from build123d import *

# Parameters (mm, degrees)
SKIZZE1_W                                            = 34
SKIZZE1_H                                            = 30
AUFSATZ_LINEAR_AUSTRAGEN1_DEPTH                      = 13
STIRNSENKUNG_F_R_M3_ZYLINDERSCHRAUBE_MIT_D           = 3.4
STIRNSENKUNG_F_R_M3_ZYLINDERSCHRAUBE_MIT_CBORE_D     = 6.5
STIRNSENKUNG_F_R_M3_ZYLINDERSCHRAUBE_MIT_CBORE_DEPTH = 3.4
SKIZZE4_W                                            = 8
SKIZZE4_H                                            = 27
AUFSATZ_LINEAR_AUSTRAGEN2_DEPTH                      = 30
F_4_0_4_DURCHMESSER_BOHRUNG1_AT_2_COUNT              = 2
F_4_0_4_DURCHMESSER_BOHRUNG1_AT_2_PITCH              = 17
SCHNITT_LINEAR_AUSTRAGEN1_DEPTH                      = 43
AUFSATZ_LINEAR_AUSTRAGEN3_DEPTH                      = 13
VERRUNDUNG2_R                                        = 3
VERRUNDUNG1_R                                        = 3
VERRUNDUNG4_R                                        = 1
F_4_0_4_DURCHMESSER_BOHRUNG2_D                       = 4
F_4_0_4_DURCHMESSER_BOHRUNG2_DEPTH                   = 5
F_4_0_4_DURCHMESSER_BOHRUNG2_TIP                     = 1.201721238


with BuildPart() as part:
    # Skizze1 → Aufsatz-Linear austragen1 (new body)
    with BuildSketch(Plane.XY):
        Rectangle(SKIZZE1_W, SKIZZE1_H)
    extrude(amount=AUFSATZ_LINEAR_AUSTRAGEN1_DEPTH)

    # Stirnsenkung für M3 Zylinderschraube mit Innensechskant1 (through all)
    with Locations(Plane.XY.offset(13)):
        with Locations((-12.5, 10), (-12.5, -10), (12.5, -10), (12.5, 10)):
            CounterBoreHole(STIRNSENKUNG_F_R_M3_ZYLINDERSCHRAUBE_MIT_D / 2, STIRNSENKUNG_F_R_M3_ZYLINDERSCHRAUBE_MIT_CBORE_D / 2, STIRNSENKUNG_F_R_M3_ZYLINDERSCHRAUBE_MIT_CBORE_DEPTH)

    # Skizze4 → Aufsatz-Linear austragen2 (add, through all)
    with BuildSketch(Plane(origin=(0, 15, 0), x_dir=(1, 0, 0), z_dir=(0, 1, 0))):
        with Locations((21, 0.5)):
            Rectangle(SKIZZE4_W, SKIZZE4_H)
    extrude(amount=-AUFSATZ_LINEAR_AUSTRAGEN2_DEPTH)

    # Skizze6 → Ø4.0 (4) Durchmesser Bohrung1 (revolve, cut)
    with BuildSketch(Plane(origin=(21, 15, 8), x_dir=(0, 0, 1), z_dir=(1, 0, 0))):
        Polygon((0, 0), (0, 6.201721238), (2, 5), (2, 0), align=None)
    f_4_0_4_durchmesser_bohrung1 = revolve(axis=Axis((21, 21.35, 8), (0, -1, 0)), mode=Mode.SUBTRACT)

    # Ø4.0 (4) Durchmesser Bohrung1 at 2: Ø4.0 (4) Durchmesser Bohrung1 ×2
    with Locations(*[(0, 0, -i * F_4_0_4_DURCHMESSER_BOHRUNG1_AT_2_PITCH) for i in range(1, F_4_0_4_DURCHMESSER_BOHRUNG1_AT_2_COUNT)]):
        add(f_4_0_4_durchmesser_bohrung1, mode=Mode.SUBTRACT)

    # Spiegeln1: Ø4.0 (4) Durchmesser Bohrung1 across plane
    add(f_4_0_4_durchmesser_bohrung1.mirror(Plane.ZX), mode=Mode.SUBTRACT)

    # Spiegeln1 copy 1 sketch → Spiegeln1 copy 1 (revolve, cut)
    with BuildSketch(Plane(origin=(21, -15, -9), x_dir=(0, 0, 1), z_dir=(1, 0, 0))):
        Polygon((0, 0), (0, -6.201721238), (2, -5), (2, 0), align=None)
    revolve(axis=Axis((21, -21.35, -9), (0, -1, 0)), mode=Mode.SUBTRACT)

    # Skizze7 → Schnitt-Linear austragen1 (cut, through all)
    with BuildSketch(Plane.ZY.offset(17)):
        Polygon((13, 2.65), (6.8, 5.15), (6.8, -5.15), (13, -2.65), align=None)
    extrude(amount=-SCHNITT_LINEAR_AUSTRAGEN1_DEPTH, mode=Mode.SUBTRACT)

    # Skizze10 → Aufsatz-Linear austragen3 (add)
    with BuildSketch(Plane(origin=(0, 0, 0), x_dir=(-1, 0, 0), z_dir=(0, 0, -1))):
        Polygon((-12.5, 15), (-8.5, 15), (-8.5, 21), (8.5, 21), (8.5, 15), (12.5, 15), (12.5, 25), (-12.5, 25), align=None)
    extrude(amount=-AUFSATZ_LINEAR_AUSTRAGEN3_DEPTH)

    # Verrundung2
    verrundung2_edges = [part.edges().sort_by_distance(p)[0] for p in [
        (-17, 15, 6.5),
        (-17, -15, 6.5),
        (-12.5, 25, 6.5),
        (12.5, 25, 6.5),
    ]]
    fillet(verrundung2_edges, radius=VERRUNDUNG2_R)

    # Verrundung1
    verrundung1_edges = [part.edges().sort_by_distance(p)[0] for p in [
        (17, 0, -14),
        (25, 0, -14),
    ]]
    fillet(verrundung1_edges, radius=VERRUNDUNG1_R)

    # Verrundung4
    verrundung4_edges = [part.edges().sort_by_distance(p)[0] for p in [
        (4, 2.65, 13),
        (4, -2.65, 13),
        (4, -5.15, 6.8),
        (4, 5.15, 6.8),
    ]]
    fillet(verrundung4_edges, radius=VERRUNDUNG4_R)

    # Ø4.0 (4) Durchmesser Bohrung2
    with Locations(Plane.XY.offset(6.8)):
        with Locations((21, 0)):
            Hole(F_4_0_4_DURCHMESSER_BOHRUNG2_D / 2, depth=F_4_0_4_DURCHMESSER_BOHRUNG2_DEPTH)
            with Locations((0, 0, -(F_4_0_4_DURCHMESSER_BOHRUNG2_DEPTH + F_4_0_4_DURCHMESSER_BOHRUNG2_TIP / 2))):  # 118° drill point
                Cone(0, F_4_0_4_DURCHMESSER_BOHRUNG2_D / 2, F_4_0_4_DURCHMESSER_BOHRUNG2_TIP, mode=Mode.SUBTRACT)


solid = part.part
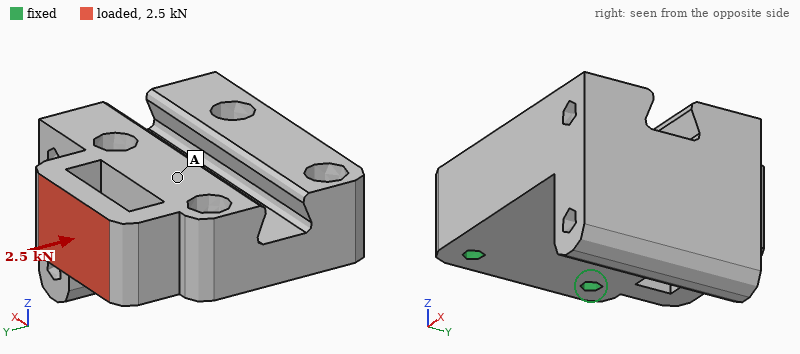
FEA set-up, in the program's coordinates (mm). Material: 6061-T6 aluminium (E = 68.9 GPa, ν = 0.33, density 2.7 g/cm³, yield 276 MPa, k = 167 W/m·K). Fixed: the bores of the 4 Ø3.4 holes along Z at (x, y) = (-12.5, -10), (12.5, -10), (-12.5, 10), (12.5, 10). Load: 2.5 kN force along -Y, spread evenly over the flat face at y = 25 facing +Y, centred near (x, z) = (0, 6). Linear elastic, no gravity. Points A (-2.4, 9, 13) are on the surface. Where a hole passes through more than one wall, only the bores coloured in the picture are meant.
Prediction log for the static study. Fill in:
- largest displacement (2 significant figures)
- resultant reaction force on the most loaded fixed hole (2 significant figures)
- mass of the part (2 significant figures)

29 µm
1.3 kN
49 g
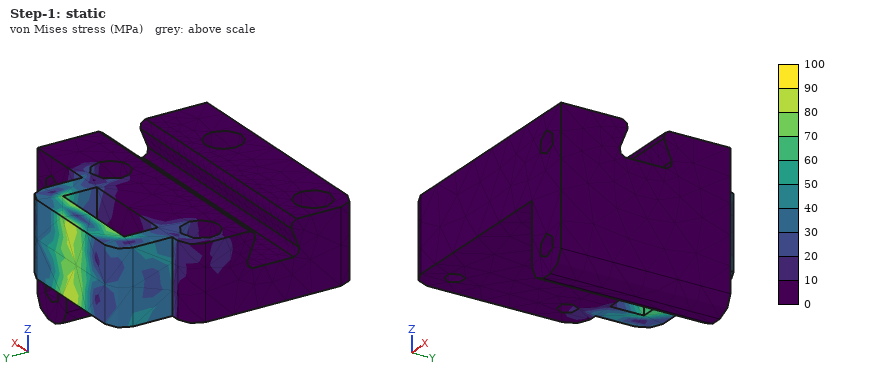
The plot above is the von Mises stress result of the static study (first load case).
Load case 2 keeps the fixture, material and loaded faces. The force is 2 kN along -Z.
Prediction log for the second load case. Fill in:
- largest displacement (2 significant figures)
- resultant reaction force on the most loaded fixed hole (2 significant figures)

49 µm
1.2 kN
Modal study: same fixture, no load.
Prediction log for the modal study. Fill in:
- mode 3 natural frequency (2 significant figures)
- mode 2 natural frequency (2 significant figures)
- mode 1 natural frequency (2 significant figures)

21 kHz
21 kHz
14 kHz
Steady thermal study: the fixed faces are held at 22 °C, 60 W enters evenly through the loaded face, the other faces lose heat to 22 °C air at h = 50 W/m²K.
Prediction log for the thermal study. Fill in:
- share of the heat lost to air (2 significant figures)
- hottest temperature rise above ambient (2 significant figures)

3.2 %
52 K
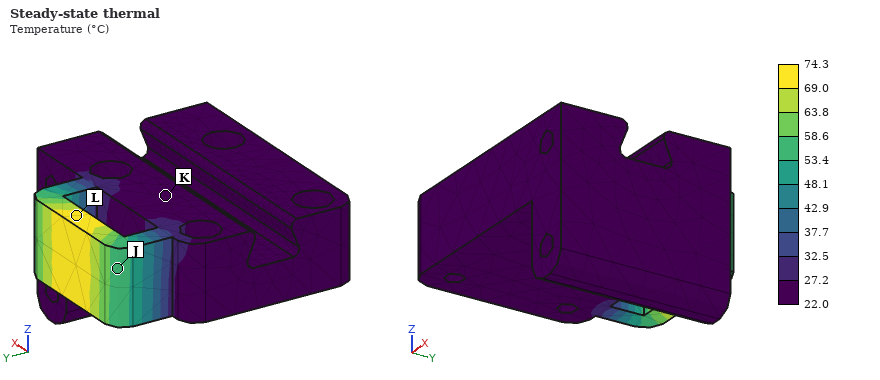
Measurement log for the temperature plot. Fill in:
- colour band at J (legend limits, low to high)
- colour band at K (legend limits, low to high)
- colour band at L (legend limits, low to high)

53.4 to 58.6 °C
22.0 to 27.2 °C
69.0 to 74.3 °C
